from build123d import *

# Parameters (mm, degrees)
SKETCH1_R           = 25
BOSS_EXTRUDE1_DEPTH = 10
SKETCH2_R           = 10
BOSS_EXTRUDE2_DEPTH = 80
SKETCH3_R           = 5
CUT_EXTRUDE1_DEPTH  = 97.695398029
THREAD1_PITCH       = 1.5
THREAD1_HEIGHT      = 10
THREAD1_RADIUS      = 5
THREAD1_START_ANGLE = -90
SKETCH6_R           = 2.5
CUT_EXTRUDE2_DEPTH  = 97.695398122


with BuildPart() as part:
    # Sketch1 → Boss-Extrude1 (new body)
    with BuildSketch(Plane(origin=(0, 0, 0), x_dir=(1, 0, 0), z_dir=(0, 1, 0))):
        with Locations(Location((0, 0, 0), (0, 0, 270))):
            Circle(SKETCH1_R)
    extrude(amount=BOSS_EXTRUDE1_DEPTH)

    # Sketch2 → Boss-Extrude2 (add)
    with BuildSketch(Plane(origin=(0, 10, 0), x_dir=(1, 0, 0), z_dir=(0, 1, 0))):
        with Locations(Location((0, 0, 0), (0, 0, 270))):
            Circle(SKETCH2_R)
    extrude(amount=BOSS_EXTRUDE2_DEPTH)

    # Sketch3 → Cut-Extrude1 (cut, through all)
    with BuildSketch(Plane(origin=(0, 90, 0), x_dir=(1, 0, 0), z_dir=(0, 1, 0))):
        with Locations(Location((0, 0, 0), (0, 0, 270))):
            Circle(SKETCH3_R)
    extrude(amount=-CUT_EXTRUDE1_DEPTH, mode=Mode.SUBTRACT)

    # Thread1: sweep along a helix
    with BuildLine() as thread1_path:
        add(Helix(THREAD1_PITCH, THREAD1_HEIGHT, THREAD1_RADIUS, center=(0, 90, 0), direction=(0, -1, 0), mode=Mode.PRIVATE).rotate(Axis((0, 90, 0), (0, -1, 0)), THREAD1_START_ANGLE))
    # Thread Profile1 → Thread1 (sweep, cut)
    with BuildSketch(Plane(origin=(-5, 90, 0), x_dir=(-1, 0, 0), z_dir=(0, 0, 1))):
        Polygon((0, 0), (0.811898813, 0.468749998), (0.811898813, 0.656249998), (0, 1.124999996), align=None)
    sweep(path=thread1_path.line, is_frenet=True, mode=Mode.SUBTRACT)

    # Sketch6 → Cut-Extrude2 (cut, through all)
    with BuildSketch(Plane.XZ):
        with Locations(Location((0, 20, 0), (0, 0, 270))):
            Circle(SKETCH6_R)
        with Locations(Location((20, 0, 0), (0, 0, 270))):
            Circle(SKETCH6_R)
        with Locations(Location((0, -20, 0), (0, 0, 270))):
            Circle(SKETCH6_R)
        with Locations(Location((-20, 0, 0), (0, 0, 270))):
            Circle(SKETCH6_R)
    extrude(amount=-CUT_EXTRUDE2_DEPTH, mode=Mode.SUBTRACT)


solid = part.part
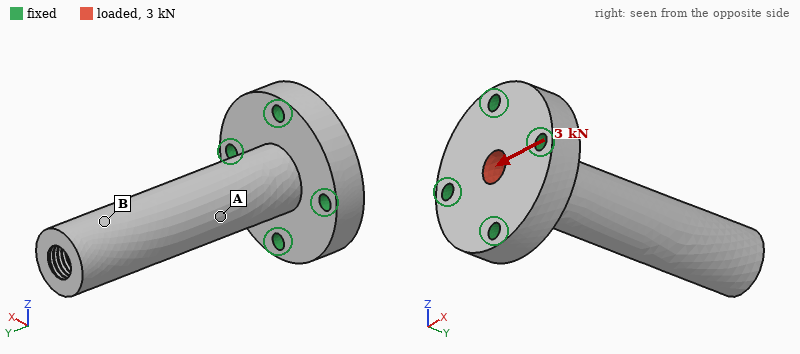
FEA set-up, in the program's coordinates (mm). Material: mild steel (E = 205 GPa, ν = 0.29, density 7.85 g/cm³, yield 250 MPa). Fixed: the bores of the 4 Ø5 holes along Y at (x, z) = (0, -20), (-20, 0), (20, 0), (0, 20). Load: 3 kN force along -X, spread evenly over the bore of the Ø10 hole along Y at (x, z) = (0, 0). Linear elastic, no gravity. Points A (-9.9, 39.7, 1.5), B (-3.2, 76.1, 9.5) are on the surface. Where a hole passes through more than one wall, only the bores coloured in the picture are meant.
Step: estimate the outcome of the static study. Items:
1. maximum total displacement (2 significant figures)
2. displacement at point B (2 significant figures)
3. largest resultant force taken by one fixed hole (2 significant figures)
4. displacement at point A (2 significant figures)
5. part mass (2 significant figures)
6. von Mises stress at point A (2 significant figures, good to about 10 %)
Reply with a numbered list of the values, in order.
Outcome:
1. 0.14 mm
2. 0.11 mm
3. 3.1 kN
4. 0.044 mm
5. 290 g
6. 41 MPa
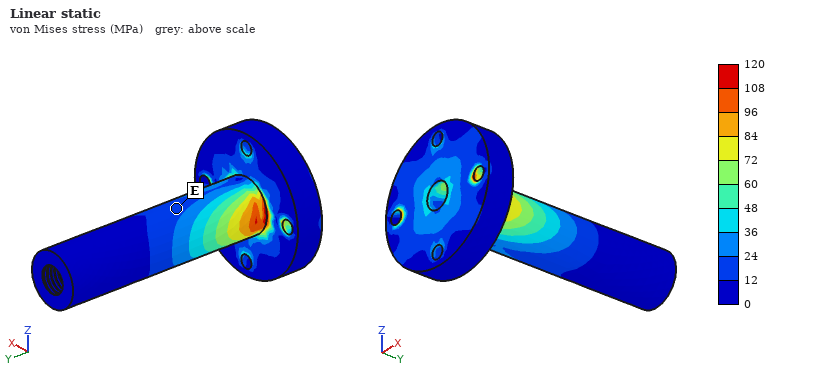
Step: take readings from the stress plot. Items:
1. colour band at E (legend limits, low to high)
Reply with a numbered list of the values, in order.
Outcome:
1. 12 to 24 MPa
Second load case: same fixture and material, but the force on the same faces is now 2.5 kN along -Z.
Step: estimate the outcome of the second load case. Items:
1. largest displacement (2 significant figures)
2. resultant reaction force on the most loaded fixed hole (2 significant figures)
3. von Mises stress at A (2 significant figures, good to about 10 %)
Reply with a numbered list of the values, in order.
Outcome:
1. 0.11 mm
2. 2.6 kN
3. 15 MPa
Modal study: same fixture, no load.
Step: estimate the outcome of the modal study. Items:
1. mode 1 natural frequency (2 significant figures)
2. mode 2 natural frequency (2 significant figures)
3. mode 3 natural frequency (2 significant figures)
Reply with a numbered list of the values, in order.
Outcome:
1. 2000 Hz
2. 2000 Hz
3. 9600 Hz
